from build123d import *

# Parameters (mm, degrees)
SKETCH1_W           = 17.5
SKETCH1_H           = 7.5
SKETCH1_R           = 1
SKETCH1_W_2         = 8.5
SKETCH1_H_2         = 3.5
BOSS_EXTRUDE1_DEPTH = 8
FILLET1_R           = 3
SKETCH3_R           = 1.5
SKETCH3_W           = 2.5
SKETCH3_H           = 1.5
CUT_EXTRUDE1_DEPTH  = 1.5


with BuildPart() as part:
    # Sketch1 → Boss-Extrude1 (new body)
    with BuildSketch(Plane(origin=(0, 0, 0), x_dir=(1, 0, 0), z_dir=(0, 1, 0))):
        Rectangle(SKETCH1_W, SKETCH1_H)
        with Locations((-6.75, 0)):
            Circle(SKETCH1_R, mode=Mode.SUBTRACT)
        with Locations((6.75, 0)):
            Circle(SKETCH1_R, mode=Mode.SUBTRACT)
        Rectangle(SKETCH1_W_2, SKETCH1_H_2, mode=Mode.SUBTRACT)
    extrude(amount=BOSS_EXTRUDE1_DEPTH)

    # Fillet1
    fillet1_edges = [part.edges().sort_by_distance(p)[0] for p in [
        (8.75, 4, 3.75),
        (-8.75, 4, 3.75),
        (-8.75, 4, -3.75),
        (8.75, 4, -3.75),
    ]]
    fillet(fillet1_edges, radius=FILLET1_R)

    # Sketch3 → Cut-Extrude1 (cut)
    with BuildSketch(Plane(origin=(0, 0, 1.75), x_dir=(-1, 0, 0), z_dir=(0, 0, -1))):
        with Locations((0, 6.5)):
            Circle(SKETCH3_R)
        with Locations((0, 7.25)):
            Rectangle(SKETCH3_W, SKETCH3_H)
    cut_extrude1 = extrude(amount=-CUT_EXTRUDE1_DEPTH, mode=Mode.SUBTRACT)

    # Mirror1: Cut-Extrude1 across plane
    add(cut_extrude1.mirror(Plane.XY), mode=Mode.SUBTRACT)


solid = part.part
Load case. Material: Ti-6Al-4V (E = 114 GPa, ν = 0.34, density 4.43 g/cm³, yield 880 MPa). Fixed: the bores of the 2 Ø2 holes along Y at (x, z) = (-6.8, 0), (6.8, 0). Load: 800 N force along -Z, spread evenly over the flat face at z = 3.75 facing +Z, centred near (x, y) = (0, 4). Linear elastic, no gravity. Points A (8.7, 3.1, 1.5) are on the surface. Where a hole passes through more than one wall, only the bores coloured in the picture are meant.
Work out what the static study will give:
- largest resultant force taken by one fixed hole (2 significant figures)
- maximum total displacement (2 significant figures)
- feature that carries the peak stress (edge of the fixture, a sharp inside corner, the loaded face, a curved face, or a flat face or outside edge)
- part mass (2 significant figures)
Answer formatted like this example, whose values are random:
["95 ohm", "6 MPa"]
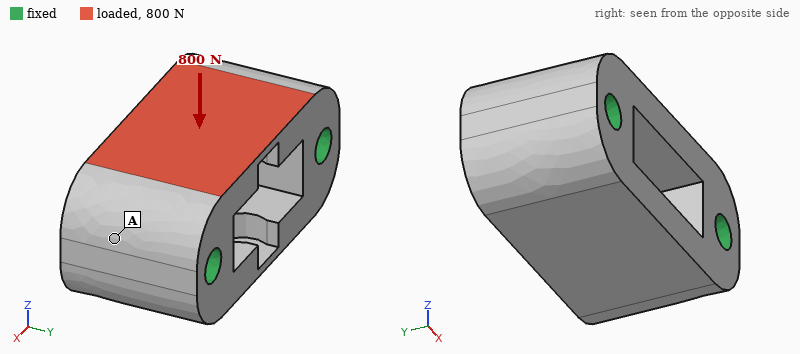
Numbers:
["450 N", "8.1 µm", "the loaded face", "3.0 g"]
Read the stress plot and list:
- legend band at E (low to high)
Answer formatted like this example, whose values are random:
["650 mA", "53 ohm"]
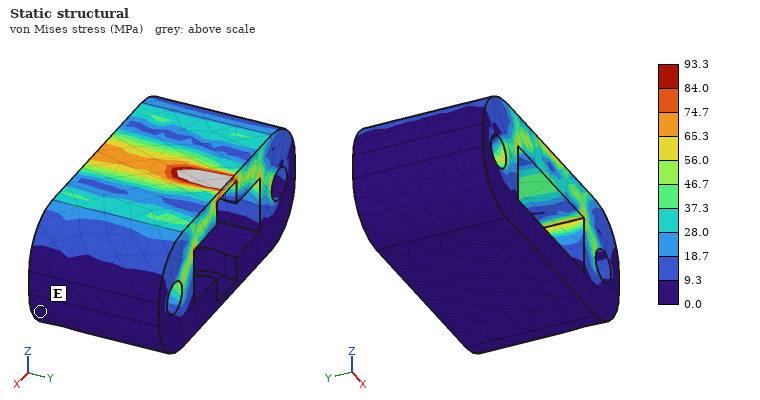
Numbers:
["0.0 to 9.3 MPa"]
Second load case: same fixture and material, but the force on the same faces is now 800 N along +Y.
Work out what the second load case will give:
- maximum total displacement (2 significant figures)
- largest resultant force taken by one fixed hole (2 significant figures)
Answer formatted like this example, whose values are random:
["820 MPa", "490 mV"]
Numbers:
["6.1 µm", "400 N"]
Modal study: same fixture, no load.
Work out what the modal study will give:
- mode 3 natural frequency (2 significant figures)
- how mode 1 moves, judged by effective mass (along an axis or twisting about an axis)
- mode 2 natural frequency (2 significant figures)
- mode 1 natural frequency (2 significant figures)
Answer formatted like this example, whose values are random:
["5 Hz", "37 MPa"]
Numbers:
["99 kHz", "along Z", "82 kHz", "78 kHz"]
